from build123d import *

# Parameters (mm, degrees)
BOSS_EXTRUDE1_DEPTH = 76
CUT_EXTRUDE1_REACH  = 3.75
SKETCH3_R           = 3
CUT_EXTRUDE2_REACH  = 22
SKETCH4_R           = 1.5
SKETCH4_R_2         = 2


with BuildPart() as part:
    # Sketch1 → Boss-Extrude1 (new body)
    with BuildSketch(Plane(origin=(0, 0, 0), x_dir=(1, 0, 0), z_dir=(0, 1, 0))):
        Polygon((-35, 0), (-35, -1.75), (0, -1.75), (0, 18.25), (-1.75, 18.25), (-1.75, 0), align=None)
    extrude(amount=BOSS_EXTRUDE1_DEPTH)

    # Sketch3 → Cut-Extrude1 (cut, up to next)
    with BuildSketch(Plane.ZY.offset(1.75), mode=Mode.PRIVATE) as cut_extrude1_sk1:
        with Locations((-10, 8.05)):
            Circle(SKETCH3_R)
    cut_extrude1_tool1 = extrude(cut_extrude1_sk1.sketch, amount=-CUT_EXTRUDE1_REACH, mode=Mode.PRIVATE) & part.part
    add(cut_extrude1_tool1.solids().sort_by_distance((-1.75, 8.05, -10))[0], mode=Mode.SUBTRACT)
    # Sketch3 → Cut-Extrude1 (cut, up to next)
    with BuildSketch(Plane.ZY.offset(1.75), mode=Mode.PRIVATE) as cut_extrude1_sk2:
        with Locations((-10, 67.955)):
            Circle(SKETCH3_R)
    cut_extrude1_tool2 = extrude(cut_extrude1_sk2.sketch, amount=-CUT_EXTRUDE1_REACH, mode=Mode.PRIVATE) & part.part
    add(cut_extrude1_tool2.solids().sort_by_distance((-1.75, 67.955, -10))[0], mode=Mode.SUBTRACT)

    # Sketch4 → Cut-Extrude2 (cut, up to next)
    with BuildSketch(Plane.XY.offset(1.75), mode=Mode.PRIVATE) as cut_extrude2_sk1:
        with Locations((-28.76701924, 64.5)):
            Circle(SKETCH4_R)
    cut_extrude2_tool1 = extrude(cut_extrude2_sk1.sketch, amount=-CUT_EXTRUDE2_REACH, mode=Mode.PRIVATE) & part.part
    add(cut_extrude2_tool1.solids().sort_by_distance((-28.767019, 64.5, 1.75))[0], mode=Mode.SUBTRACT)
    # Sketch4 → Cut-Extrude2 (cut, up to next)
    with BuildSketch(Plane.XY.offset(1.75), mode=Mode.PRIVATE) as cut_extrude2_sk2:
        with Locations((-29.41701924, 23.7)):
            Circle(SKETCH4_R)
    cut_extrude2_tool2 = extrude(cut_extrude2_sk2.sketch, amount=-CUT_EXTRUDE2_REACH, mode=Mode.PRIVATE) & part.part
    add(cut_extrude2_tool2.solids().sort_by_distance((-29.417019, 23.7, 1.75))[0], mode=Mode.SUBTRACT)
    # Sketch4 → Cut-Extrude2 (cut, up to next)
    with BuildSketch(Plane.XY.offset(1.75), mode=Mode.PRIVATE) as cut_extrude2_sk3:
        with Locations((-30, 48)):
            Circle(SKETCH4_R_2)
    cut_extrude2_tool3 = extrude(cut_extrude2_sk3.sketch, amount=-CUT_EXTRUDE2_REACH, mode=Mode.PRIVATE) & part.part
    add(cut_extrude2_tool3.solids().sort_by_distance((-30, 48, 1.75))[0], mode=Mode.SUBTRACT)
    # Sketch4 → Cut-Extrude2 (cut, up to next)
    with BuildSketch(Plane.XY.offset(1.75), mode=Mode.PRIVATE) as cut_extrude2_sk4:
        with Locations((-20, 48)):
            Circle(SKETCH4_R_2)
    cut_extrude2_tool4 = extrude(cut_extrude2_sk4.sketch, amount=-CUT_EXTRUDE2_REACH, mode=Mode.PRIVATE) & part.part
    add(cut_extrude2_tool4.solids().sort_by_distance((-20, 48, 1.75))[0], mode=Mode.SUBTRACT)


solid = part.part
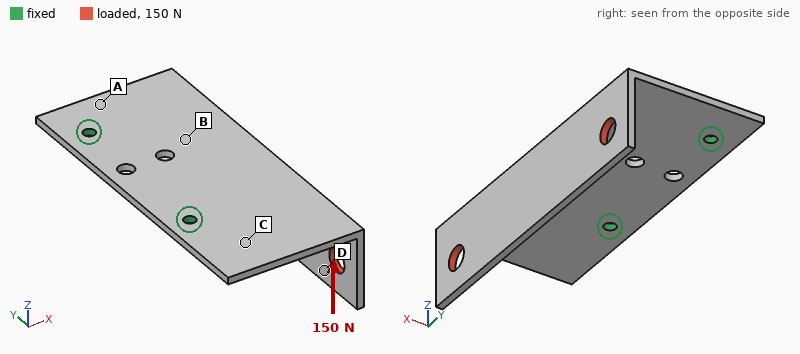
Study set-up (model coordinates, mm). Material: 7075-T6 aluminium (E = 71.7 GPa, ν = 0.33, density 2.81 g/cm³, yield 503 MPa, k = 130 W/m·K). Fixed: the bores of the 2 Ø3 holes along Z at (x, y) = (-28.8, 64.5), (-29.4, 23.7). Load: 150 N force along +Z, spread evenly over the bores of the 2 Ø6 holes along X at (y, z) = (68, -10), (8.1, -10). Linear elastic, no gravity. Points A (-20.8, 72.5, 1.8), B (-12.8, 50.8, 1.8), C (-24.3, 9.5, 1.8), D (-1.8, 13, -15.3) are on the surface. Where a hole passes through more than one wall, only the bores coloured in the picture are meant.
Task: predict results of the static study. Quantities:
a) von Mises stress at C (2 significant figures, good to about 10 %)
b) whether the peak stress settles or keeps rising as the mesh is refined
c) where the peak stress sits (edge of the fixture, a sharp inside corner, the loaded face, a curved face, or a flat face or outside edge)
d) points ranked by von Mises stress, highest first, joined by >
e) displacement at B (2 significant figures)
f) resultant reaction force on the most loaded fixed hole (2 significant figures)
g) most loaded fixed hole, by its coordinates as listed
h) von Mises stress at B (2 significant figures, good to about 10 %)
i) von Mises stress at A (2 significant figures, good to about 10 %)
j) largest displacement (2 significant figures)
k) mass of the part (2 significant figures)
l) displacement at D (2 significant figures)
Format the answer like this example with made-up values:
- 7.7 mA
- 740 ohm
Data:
- 61 MPa
- keeps rising
- edge of the fixture
- A > C > B > D
- 0.28 mm
- 93 N
- (-29.4, 23.7)
- 39 MPa
- 90 MPa
- 0.97 mm
- 19 g
- 0.84 mm
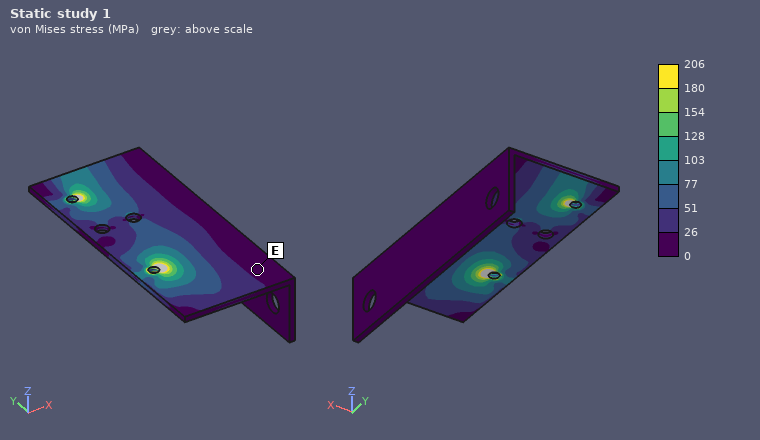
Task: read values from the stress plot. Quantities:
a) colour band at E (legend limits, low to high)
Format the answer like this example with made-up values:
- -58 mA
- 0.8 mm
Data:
- 0 to 26 MPa
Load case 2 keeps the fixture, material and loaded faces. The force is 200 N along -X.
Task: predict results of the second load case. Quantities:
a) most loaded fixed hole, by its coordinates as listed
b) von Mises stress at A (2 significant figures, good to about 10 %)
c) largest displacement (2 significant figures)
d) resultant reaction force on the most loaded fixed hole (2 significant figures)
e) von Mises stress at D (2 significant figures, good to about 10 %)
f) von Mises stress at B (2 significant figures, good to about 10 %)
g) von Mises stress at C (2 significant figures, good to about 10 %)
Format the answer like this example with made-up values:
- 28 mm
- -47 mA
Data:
- (-29.4, 23.7)
- 65 MPa
- 0.85 mm
- 130 N
- 16 MPa
- 45 MPa
- 42 MPa
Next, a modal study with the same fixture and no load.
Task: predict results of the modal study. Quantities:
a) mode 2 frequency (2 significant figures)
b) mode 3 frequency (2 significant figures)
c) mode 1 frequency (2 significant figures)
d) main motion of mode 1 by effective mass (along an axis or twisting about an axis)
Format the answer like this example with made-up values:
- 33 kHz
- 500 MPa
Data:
- 1100 Hz
- 2500 Hz
- 710 Hz
- along Z
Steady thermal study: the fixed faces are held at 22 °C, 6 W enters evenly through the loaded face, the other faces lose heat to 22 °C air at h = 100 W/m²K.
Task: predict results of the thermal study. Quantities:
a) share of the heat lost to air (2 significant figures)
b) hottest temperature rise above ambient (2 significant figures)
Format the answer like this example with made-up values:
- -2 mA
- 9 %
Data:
- 64 %
- 13 K
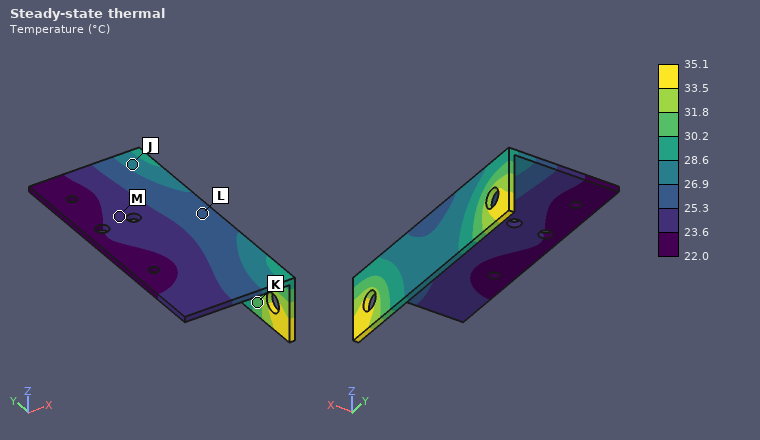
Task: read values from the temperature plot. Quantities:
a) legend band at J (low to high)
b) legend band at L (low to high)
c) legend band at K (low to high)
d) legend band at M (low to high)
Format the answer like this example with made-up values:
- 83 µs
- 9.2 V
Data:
- 26.9 to 28.6 °C
- 25.3 to 26.9 °C
- 30.2 to 31.8 °C
- 23.6 to 25.3 °C
